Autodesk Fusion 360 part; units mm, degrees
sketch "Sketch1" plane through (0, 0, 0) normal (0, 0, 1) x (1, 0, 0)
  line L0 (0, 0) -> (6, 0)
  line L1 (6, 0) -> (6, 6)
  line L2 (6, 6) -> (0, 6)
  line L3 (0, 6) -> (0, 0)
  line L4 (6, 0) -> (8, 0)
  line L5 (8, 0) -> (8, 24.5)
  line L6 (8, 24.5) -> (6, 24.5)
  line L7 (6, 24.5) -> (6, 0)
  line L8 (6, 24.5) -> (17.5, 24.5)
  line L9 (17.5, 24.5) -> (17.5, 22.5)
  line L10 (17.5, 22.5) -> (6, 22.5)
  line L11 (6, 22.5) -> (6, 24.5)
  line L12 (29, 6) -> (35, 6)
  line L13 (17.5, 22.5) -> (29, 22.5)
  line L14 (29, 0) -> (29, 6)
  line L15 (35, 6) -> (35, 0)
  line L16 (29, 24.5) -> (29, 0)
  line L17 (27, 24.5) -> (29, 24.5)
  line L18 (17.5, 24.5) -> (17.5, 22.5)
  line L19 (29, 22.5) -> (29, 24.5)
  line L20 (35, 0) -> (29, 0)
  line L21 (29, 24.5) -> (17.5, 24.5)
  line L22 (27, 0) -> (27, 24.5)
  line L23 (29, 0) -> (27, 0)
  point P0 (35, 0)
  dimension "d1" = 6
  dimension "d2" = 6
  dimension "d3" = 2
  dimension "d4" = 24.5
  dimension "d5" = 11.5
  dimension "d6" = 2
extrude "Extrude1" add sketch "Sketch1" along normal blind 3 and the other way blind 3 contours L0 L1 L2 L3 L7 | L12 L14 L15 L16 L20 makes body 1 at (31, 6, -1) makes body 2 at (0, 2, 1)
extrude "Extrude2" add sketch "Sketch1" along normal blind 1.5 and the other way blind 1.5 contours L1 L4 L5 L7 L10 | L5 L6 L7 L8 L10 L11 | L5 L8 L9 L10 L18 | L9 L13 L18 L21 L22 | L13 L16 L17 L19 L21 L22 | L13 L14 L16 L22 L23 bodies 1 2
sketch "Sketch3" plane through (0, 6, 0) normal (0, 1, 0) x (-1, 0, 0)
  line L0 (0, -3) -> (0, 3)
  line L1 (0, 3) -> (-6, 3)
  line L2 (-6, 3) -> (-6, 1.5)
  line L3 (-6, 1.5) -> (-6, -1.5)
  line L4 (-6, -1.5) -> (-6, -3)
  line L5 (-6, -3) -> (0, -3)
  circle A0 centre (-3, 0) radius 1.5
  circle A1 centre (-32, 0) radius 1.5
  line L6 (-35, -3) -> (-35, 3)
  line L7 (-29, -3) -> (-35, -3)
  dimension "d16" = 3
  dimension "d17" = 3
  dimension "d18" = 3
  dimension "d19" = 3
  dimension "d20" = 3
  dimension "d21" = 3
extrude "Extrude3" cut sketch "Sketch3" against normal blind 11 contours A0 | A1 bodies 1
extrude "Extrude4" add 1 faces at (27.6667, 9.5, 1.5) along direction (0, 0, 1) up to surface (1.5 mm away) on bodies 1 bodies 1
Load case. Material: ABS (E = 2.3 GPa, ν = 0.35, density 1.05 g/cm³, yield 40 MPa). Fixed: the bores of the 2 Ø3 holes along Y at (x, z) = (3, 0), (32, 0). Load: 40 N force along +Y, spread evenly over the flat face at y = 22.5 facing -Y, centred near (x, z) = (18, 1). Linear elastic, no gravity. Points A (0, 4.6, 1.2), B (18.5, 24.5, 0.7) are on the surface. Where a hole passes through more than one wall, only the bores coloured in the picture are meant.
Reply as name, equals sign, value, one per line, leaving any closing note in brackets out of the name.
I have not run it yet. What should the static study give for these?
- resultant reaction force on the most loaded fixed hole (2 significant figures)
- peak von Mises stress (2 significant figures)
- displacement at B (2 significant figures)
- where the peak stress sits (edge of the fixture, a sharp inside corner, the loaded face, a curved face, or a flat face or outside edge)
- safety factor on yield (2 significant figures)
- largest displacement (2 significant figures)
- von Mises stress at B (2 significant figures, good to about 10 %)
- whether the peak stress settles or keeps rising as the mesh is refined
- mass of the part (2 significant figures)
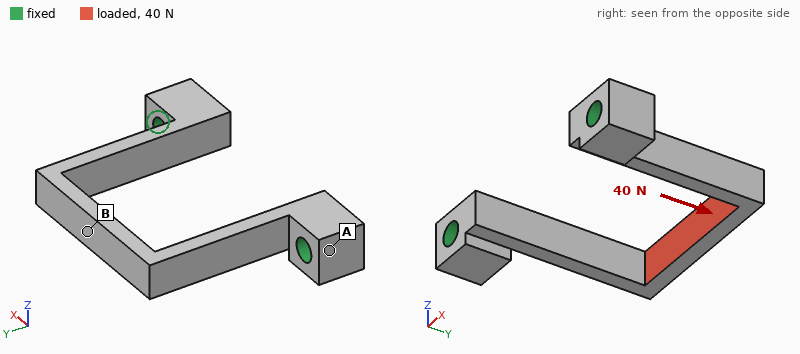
resultant reaction force on the most loaded fixed hole = 21 N
peak von Mises stress = 20 MPa
displacement at B = 0.34 mm
where the peak stress sits = a flat face or outside edge
safety factor on yield = 2.0
largest displacement = 0.35 mm
von Mises stress at B = 19 MPa
whether the peak stress settles or keeps rising as the mesh is refined = settles
mass of the part = 1.0 g
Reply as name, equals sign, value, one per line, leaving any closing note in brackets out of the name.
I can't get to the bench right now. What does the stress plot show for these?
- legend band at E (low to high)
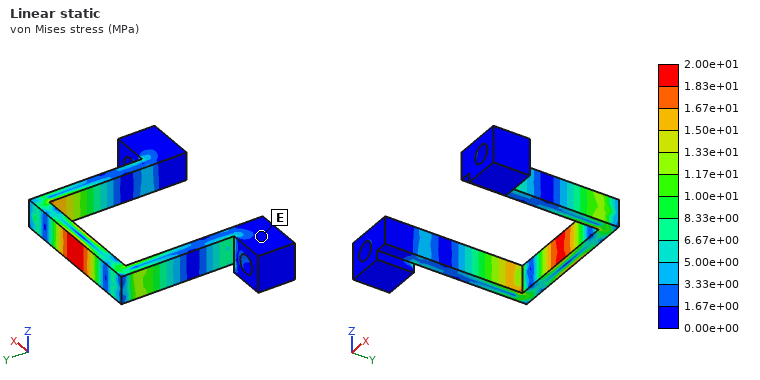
legend band at E = 0.00e+00 to 1.67e+00 MPa
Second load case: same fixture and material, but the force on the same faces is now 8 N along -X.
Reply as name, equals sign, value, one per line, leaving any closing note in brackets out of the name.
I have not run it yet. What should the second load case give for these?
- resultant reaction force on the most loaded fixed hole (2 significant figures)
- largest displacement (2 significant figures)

resultant reaction force on the most loaded fixed hole = 4.8 N
largest displacement = 0.45 mm
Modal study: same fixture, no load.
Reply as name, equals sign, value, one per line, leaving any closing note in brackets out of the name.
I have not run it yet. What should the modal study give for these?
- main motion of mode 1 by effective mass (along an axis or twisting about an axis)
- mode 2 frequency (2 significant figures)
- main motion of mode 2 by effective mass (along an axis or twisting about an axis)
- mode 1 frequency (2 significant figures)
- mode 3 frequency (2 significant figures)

main motion of mode 1 by effective mass = along X
mode 2 frequency = 1500 Hz
main motion of mode 2 by effective mass = along Z
mode 1 frequency = 1200 Hz
mode 3 frequency = 2400 Hz
